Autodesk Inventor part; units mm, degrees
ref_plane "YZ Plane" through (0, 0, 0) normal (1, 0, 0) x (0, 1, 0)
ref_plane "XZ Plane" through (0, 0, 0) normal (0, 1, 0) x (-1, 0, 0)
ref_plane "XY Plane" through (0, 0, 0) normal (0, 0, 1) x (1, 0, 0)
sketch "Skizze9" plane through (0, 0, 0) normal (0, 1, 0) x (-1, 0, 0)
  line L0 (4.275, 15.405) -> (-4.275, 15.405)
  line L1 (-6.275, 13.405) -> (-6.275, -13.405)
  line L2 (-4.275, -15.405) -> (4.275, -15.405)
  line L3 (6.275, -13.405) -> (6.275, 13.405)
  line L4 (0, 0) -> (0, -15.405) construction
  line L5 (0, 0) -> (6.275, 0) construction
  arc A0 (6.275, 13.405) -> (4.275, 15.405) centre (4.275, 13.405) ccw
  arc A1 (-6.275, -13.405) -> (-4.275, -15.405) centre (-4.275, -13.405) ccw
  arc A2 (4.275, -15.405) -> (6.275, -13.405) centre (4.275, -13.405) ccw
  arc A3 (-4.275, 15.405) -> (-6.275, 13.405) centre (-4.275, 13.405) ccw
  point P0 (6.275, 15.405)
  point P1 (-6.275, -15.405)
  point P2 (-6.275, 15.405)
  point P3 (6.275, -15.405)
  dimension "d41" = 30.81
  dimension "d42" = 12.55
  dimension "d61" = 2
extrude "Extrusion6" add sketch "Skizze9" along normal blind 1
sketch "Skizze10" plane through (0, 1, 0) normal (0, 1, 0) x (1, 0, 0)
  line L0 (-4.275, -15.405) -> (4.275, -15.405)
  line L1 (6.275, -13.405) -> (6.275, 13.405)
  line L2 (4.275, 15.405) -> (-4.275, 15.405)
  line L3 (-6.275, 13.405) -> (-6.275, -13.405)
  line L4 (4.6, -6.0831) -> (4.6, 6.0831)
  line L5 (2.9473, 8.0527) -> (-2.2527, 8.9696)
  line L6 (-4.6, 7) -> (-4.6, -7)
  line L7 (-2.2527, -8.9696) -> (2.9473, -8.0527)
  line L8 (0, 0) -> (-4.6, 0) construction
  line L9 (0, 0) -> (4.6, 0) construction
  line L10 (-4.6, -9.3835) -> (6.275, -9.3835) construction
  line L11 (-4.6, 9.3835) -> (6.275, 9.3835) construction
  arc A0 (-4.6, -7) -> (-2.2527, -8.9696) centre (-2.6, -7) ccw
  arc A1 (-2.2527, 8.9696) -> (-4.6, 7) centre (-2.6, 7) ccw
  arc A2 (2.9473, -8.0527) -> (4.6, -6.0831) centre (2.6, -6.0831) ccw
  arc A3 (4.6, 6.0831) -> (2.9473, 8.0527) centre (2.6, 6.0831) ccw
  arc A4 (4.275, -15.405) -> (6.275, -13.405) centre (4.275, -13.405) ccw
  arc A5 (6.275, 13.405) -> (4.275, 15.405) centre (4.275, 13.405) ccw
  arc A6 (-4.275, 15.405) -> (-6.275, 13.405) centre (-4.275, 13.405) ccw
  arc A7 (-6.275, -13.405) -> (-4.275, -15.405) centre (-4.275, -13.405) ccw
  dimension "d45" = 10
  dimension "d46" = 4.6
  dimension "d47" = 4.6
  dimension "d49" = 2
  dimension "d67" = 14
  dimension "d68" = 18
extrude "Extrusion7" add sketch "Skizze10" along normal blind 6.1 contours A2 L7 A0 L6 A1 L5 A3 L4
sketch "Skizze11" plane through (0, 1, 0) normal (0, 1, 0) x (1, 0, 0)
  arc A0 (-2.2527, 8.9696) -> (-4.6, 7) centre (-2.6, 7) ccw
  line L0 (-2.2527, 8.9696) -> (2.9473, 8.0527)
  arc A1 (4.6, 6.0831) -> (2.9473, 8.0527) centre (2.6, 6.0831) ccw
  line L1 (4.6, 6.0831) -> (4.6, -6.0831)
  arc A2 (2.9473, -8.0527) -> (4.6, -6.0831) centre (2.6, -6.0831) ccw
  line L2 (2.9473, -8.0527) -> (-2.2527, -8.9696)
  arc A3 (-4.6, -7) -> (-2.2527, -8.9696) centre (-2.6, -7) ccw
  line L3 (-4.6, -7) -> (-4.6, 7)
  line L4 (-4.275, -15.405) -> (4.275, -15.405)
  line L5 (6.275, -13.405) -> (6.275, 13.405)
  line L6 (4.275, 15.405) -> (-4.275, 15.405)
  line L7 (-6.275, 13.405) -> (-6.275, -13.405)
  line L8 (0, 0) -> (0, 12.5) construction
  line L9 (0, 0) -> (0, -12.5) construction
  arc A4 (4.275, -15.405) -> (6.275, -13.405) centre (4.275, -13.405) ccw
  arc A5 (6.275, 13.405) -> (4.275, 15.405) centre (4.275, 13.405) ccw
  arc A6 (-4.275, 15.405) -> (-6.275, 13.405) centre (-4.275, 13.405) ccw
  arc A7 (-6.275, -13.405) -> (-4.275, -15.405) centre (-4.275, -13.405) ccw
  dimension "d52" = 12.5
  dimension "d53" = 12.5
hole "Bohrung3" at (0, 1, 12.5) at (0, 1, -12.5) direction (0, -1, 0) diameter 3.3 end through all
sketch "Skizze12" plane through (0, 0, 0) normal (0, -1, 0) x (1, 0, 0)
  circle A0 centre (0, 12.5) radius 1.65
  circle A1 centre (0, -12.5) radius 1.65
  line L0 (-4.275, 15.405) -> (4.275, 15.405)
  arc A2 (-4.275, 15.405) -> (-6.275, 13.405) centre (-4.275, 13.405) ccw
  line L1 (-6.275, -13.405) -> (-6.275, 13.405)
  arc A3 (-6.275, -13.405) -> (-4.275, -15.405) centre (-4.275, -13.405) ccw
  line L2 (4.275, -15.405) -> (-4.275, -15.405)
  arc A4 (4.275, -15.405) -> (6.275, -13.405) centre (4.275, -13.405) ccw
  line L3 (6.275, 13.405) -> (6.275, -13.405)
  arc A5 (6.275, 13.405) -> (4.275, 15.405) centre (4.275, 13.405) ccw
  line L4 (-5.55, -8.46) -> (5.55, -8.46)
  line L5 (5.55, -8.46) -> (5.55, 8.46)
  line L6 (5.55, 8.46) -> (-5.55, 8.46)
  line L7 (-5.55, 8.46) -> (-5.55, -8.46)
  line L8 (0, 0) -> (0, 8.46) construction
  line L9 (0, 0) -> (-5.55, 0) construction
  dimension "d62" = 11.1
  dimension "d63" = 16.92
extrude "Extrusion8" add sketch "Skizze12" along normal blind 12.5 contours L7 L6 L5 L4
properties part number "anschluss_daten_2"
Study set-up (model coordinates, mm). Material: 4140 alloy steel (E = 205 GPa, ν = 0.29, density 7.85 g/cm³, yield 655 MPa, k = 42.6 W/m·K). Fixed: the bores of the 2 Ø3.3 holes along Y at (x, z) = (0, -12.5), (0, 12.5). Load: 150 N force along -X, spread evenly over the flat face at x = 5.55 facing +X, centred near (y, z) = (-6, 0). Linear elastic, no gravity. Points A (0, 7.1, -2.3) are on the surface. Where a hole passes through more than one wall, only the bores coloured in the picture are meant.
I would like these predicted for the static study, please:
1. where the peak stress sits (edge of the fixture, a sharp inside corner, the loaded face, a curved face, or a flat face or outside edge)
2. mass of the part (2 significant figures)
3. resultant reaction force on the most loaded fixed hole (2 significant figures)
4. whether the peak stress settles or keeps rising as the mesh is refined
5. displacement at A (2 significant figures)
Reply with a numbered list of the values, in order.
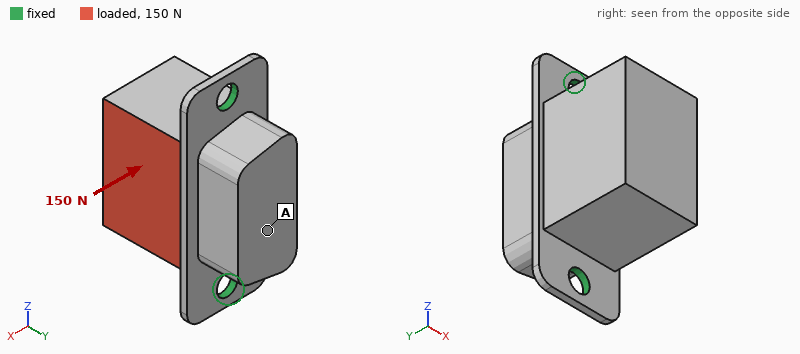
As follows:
1. edge of the fixture
2. 29 g
3. 77 N
4. keeps rising
5. 16 µm
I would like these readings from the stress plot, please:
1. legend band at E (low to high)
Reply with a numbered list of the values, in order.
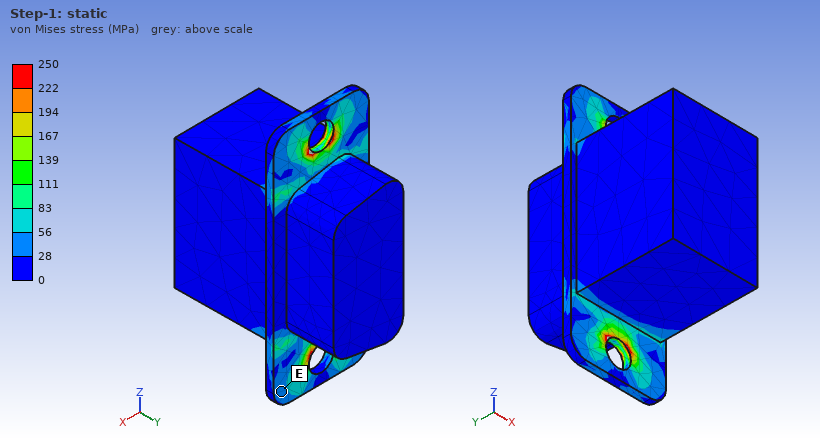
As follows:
1. 28 to 56 MPa
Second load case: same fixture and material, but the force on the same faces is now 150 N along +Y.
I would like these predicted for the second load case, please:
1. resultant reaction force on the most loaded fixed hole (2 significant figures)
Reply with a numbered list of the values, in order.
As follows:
1. 76 N
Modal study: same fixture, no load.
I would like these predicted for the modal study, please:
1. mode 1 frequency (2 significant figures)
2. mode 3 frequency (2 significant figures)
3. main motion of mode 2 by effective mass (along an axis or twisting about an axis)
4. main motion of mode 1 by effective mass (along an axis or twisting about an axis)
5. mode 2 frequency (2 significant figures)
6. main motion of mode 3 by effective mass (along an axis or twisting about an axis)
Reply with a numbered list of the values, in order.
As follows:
1. 2600 Hz
2. 10 kHz
3. along Y
4. along X
5. 8700 Hz
6. along Z
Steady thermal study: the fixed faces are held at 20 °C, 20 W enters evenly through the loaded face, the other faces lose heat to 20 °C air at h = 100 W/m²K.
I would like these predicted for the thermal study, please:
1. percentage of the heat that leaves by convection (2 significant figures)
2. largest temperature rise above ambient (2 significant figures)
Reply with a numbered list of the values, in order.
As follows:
1. 41 %
2. 77 K
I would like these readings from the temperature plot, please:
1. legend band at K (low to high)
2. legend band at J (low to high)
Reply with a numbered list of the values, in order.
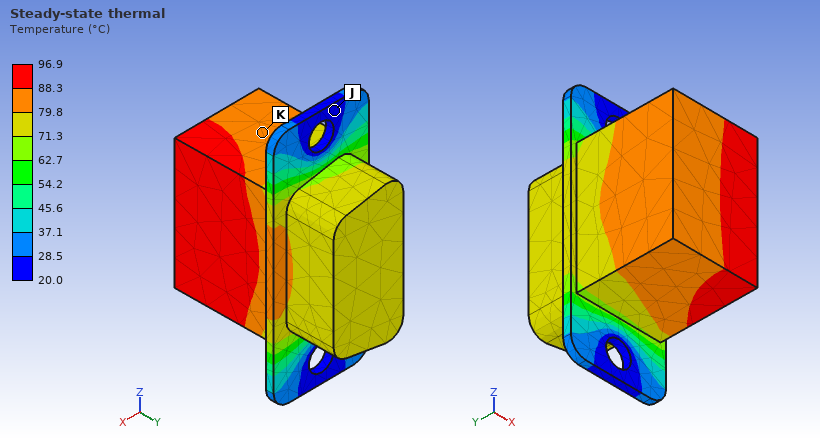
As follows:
1. 79.8 to 88.3 °C
2. 20.0 to 28.5 °C
